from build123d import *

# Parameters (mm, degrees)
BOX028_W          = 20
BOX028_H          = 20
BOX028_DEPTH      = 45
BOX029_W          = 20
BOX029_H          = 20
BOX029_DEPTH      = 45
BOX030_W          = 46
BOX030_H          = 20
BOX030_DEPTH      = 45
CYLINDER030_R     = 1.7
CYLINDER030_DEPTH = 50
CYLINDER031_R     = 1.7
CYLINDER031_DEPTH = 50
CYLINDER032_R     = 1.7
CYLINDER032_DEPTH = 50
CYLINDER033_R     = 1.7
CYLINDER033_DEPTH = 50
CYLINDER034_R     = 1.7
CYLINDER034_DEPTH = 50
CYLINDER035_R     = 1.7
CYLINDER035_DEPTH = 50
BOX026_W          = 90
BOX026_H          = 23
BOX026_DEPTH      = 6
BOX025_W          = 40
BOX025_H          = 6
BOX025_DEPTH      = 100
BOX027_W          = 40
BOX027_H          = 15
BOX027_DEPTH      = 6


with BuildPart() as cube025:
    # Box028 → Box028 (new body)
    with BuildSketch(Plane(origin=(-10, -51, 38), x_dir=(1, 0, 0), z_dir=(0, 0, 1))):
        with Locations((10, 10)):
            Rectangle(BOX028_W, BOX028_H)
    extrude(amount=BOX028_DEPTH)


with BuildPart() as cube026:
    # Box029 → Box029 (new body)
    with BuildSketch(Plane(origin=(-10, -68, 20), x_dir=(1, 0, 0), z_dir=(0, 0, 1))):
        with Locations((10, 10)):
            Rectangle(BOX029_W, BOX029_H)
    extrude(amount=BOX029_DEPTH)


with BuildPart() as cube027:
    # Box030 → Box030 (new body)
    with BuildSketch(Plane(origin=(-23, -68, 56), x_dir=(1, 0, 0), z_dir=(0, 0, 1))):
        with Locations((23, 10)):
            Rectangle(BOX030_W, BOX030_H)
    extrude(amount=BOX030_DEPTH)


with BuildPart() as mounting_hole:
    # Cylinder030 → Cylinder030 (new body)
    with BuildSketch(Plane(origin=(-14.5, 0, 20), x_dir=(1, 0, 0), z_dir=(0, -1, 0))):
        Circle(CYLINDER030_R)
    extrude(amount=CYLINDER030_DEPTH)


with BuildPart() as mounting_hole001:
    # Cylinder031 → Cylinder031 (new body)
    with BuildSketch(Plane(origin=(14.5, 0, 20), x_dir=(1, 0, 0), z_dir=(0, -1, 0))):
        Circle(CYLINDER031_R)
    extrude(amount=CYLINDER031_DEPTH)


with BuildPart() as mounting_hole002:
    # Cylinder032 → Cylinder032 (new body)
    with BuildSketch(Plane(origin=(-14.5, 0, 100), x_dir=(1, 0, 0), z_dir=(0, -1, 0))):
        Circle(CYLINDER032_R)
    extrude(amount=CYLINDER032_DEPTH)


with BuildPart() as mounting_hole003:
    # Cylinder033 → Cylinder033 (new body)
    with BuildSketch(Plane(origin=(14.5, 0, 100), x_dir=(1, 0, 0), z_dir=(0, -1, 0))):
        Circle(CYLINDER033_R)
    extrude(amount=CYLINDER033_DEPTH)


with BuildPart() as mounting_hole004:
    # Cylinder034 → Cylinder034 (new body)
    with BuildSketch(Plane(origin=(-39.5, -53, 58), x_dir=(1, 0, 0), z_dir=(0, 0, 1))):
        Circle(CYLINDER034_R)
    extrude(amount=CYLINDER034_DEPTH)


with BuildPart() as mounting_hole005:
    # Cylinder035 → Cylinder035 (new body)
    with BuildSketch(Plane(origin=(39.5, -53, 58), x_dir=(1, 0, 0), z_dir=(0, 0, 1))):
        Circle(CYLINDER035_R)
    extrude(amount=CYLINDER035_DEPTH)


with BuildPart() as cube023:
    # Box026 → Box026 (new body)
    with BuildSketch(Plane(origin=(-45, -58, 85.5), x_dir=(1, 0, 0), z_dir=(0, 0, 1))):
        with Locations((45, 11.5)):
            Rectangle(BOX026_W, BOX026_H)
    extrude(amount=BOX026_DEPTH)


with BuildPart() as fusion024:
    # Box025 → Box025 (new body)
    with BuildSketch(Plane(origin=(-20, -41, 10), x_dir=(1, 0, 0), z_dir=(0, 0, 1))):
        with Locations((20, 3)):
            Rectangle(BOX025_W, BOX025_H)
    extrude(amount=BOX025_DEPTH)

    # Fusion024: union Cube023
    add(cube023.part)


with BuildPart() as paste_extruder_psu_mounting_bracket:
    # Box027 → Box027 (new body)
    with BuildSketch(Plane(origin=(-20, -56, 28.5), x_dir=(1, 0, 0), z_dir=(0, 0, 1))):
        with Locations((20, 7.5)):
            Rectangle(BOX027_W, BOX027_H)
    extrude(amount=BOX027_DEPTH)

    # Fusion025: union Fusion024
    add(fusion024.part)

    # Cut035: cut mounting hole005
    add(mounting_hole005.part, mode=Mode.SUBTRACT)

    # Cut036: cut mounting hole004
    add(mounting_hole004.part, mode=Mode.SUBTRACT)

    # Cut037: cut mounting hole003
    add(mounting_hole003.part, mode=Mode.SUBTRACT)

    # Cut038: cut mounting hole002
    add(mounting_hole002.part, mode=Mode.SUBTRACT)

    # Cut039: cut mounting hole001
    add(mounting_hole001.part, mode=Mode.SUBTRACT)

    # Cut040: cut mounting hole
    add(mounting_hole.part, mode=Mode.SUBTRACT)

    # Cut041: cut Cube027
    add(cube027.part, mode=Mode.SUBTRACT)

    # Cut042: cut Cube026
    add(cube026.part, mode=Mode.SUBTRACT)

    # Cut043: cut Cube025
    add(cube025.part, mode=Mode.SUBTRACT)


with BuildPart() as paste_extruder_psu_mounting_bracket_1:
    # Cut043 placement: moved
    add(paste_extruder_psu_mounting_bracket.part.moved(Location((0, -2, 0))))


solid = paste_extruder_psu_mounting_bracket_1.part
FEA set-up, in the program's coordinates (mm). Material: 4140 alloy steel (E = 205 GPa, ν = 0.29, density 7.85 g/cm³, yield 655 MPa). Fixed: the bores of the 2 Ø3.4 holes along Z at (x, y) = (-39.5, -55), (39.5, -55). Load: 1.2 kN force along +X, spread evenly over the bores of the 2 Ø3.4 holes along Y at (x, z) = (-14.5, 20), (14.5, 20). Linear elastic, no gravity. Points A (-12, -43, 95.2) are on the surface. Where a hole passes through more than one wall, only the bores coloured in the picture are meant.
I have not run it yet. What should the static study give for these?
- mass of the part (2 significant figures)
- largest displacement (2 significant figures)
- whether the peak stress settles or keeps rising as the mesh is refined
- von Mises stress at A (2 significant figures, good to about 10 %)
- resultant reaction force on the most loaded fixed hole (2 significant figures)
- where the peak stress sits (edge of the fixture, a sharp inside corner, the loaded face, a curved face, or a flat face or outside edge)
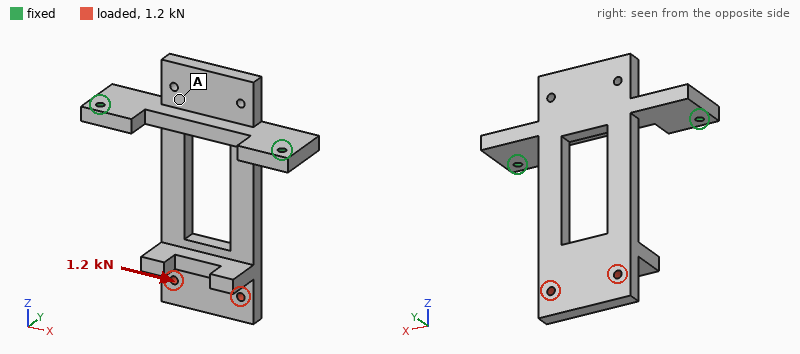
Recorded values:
230 g
0.25 mm
keeps rising
28 MPa
1.5 kN
edge of the fixture
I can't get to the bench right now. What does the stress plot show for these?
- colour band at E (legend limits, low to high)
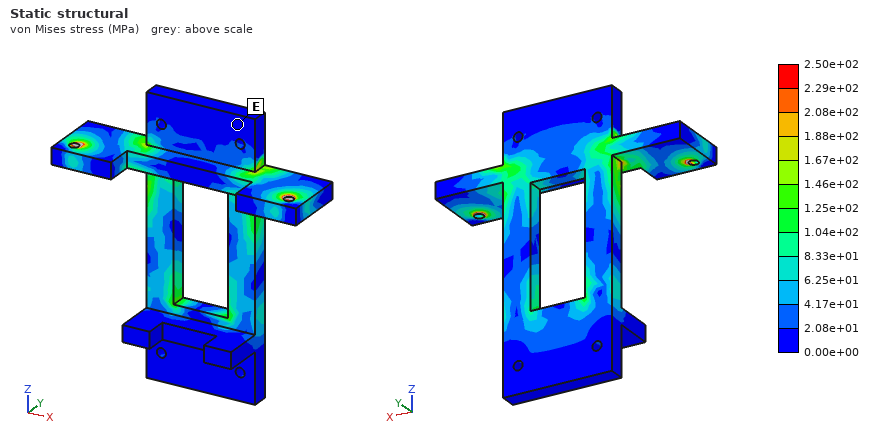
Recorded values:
0.00e+00 to 2.08e+01 MPa
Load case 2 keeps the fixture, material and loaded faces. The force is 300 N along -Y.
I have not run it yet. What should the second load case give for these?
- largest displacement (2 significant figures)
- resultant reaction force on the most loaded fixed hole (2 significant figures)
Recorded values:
0.80 mm
280 N
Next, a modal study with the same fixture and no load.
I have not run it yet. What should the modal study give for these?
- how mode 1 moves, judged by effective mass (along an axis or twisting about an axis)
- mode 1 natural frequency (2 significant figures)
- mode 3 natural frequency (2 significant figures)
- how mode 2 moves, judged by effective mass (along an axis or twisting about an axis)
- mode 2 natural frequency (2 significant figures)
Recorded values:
along Y
420 Hz
2000 Hz
along X
1300 Hz
